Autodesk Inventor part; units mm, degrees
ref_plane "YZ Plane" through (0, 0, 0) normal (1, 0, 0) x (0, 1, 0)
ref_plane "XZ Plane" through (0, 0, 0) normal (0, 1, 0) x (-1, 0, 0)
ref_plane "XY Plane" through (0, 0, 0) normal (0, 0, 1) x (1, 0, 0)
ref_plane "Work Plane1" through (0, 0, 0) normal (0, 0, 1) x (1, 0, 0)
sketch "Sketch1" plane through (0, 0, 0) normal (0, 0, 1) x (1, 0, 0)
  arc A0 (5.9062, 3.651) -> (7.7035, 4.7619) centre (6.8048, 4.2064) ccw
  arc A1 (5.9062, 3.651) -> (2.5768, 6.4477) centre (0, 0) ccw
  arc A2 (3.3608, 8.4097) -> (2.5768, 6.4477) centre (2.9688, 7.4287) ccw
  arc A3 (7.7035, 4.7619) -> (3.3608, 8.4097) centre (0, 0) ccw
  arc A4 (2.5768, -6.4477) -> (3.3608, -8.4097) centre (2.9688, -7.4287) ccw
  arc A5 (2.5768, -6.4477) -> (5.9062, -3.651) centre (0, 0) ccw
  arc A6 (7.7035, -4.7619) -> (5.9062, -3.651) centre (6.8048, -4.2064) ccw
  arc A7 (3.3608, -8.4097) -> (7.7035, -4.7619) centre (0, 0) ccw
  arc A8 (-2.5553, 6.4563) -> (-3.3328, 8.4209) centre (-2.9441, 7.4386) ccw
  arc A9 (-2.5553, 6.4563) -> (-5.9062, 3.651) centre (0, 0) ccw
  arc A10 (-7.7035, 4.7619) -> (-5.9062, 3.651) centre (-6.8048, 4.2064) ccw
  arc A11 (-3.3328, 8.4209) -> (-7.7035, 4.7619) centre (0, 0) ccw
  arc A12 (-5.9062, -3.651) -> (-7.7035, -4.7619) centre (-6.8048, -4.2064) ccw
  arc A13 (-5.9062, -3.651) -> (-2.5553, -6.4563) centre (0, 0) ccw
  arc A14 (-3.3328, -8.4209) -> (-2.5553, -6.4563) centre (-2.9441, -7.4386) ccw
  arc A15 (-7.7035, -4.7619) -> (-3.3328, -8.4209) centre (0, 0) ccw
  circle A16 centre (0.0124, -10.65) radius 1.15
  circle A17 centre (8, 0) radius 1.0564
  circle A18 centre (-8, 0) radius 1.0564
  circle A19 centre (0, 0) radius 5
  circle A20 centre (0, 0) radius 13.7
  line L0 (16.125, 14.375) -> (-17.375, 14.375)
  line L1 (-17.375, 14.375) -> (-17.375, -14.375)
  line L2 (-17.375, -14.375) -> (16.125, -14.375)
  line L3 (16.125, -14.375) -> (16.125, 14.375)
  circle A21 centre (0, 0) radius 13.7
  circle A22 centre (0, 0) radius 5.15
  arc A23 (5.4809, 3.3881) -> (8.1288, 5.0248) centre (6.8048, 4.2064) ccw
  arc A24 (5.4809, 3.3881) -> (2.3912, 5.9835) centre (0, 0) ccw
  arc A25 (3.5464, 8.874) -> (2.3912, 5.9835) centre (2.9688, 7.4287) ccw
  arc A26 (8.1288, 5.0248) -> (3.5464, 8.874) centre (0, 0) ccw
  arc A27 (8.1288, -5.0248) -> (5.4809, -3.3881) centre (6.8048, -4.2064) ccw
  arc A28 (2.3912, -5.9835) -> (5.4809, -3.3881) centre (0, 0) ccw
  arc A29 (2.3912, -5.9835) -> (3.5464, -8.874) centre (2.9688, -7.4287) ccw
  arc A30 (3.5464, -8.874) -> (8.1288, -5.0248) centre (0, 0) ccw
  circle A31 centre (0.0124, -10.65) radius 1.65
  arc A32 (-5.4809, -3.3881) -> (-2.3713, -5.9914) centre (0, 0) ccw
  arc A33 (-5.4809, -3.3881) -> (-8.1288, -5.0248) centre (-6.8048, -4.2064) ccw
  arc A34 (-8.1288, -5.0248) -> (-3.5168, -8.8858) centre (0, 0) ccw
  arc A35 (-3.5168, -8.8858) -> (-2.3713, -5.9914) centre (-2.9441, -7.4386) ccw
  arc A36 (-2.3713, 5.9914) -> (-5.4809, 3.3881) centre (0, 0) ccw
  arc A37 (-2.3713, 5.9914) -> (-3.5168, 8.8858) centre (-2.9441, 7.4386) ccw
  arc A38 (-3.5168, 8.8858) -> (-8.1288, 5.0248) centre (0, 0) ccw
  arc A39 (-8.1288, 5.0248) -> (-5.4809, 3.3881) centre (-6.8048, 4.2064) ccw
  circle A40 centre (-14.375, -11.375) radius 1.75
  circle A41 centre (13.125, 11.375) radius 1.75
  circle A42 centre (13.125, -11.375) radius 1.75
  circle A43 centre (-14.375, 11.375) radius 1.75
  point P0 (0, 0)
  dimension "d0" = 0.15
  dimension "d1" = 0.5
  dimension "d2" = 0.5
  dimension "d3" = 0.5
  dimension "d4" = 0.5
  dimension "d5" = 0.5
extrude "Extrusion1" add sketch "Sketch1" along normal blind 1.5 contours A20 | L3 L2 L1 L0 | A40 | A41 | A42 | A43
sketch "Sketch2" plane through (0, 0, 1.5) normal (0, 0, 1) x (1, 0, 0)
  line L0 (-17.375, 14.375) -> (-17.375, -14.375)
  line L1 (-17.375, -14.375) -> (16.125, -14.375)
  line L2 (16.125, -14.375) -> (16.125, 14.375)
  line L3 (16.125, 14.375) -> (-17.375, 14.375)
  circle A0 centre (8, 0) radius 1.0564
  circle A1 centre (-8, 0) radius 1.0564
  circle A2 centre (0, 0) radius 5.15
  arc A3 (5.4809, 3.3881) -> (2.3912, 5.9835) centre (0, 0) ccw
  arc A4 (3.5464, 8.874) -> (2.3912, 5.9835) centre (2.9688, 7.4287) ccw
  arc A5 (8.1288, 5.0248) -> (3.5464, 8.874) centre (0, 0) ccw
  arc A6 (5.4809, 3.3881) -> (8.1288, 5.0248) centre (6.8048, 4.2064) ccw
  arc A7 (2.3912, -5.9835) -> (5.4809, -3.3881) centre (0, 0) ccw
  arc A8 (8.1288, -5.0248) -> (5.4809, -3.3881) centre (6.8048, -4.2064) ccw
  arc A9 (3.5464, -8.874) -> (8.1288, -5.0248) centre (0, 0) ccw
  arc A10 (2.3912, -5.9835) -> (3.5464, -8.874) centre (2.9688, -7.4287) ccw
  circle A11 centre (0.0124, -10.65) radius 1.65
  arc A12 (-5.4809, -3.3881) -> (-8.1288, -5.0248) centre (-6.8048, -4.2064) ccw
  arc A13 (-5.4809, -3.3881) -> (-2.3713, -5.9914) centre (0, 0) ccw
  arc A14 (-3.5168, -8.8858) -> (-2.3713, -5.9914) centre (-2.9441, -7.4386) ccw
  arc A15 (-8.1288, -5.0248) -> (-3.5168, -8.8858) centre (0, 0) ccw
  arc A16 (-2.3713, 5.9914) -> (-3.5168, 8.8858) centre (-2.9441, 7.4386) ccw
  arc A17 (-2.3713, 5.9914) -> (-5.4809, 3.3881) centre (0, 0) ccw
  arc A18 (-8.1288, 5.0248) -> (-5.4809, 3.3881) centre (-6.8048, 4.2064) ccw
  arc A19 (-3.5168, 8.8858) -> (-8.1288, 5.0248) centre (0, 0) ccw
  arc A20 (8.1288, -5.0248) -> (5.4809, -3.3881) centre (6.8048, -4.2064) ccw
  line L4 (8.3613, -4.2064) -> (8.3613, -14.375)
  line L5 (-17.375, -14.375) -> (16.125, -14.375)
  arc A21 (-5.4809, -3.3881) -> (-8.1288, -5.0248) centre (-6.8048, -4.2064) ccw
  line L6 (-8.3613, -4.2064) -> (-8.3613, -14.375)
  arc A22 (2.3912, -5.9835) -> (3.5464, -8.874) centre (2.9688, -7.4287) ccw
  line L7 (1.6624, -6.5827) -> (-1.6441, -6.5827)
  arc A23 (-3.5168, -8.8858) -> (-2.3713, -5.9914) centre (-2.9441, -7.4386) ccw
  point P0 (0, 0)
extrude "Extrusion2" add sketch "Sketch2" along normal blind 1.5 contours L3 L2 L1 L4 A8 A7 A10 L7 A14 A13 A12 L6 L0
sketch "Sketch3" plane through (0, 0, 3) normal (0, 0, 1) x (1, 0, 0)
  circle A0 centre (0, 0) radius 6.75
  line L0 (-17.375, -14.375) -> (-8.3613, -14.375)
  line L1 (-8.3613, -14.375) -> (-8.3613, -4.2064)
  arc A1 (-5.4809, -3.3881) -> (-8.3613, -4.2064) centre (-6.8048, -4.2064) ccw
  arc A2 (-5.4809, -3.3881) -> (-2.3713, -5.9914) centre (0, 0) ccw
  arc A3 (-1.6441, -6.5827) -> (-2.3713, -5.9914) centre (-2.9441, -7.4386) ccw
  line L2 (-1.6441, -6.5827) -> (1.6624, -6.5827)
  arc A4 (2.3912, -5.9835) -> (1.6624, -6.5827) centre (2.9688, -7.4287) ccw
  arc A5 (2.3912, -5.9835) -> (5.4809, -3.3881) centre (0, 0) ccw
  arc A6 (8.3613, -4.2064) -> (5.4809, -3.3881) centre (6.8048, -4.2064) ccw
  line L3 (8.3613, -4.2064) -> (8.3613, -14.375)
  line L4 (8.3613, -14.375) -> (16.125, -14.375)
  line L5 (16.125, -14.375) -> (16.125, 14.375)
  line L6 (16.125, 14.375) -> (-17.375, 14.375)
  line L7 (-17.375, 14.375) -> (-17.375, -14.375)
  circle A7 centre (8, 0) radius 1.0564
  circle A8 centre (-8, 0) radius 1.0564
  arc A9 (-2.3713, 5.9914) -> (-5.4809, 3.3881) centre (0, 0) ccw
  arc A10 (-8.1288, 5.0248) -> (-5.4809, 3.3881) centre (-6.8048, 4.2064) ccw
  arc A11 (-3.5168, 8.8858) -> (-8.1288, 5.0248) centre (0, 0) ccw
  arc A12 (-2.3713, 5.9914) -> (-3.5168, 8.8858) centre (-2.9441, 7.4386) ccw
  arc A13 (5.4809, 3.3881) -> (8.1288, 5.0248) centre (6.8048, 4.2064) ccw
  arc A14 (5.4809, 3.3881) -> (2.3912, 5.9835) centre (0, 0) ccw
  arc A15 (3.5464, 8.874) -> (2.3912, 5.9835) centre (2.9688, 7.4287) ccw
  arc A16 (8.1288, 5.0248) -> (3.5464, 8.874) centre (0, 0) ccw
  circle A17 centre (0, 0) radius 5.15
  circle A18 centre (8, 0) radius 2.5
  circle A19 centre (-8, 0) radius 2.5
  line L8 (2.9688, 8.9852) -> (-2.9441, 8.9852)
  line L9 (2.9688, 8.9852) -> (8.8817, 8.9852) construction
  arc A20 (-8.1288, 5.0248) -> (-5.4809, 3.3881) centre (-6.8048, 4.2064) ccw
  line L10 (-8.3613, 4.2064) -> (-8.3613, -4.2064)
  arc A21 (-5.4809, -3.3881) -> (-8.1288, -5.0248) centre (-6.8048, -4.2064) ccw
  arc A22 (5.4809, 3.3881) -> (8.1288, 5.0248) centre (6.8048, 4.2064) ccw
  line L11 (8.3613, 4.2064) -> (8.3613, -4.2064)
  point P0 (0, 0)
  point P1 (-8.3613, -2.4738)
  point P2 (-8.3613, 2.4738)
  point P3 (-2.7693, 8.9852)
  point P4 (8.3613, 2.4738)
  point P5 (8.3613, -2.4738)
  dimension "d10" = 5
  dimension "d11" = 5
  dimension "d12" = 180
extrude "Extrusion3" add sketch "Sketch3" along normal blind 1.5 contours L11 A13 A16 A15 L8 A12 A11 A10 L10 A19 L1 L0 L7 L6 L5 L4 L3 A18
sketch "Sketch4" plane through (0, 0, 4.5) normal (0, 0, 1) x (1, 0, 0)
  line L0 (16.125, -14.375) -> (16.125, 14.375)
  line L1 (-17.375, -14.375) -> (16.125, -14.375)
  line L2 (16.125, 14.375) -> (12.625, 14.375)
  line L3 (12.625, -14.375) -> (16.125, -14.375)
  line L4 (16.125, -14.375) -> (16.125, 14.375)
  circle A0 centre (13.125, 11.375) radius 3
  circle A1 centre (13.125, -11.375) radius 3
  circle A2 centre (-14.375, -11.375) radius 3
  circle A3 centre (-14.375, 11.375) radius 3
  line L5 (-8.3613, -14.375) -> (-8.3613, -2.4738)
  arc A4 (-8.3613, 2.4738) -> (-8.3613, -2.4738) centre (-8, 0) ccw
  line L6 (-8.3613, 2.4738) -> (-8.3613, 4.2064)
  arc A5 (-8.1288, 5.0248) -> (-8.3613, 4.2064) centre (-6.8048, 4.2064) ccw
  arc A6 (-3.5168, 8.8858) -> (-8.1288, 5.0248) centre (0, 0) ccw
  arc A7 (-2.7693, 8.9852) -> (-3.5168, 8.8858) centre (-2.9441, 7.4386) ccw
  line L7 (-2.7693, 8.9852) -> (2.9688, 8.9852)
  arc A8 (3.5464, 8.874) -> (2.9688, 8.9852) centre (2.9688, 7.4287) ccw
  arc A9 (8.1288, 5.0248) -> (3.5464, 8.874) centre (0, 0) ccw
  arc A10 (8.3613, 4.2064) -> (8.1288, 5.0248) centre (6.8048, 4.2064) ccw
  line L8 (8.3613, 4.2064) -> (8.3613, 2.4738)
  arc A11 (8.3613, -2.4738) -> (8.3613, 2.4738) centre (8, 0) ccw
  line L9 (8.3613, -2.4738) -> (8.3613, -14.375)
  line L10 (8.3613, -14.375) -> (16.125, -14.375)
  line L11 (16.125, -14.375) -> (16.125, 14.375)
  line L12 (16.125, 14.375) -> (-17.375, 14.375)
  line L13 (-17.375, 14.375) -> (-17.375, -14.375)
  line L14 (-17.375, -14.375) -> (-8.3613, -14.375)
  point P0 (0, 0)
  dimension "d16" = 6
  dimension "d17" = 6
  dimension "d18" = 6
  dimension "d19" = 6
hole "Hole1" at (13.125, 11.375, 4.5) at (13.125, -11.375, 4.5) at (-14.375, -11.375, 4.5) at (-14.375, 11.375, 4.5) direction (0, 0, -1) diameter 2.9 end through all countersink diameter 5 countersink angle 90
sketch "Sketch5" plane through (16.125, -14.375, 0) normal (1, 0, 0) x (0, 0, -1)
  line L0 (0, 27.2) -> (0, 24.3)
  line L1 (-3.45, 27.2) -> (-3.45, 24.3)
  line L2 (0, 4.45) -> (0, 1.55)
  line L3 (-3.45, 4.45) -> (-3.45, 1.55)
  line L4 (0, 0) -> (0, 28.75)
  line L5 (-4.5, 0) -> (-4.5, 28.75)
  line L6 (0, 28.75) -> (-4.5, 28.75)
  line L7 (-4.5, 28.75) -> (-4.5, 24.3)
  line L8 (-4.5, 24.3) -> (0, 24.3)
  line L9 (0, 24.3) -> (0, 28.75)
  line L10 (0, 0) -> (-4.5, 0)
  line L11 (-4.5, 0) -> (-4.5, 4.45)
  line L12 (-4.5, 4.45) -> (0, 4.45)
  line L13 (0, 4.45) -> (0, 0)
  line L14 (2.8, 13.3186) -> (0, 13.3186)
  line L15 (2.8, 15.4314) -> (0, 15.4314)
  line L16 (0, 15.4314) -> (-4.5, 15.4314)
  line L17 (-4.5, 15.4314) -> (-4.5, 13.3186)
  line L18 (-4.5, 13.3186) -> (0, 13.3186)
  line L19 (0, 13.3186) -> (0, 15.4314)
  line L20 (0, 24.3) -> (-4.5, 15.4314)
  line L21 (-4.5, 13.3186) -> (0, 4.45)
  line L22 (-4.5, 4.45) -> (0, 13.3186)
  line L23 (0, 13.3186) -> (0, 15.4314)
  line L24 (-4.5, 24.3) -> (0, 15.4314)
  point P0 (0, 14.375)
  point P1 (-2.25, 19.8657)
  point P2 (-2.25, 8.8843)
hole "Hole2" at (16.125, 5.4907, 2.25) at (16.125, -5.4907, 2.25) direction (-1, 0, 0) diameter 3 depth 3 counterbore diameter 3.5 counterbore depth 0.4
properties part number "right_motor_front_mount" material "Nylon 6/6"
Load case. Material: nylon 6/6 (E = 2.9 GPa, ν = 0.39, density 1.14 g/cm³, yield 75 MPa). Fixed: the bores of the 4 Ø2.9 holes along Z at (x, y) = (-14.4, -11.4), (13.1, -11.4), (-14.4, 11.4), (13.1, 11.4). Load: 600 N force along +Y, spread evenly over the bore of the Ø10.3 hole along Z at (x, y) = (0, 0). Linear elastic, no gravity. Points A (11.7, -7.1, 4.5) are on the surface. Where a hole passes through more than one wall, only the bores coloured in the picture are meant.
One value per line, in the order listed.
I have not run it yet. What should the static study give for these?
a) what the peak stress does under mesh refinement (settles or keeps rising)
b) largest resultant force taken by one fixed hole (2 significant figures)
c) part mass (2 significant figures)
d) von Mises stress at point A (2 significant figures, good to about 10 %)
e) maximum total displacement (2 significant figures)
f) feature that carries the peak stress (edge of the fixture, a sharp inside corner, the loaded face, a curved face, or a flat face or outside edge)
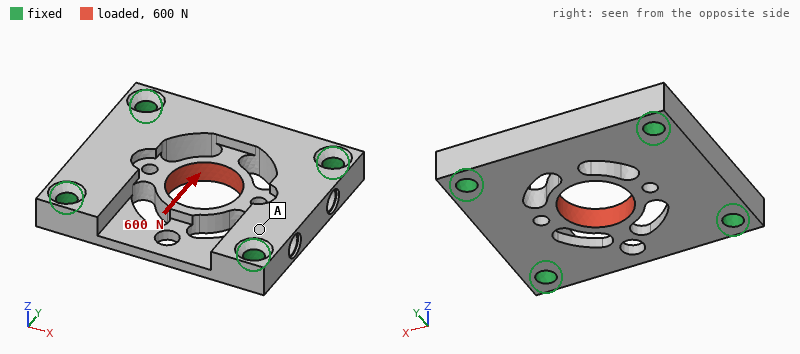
keeps rising
180 N
3.2 g
5.7 MPa
0.16 mm
a sharp inside corner
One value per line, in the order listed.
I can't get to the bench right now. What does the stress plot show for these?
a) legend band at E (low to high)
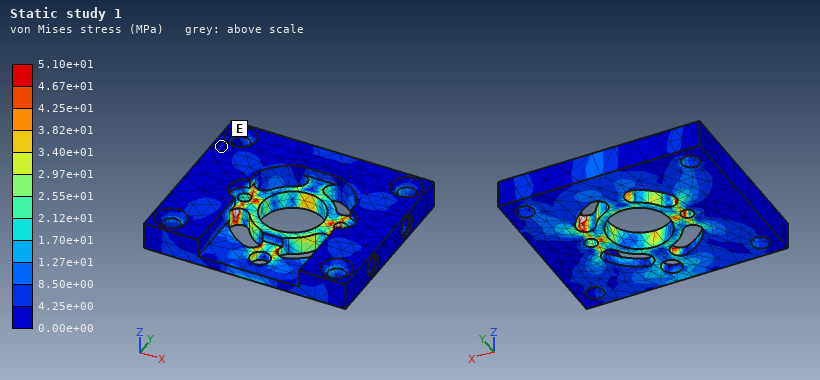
0.00e+00 to 4.25e+00 MPa
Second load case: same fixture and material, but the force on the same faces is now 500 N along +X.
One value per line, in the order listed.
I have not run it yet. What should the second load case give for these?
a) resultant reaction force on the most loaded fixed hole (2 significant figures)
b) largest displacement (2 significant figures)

160 N
0.21 mm
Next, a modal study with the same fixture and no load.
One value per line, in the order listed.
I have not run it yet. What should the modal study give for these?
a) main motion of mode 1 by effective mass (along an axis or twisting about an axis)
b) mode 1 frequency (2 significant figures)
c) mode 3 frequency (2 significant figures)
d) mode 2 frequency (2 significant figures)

along Z
6700 Hz
9800 Hz
8100 Hz
